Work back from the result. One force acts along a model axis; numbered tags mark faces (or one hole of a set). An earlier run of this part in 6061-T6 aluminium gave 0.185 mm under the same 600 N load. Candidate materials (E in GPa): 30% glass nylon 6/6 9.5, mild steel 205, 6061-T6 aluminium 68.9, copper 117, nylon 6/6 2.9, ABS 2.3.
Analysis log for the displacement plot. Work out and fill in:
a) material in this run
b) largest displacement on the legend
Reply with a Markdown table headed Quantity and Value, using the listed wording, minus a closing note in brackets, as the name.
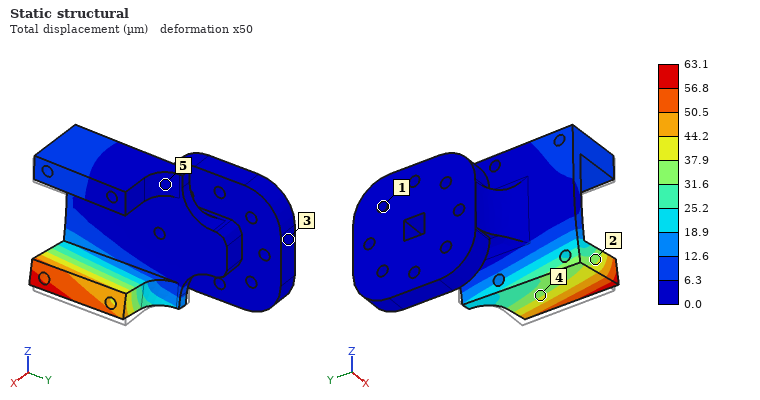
| Quantity | Value |
|---|---|
| material in this run | mild steel |
| largest displacement on the legend | 63.1 µm |
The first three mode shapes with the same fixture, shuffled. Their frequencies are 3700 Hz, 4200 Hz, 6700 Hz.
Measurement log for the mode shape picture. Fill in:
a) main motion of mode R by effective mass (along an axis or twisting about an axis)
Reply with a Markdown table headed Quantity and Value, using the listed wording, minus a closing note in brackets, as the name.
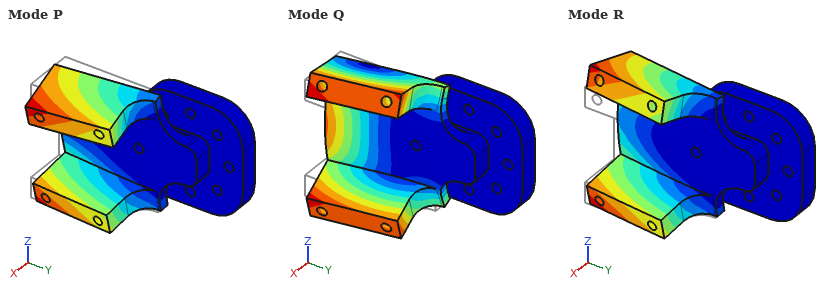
| Quantity | Value |
|---|---|
| main motion of mode R by effective mass | along X |
